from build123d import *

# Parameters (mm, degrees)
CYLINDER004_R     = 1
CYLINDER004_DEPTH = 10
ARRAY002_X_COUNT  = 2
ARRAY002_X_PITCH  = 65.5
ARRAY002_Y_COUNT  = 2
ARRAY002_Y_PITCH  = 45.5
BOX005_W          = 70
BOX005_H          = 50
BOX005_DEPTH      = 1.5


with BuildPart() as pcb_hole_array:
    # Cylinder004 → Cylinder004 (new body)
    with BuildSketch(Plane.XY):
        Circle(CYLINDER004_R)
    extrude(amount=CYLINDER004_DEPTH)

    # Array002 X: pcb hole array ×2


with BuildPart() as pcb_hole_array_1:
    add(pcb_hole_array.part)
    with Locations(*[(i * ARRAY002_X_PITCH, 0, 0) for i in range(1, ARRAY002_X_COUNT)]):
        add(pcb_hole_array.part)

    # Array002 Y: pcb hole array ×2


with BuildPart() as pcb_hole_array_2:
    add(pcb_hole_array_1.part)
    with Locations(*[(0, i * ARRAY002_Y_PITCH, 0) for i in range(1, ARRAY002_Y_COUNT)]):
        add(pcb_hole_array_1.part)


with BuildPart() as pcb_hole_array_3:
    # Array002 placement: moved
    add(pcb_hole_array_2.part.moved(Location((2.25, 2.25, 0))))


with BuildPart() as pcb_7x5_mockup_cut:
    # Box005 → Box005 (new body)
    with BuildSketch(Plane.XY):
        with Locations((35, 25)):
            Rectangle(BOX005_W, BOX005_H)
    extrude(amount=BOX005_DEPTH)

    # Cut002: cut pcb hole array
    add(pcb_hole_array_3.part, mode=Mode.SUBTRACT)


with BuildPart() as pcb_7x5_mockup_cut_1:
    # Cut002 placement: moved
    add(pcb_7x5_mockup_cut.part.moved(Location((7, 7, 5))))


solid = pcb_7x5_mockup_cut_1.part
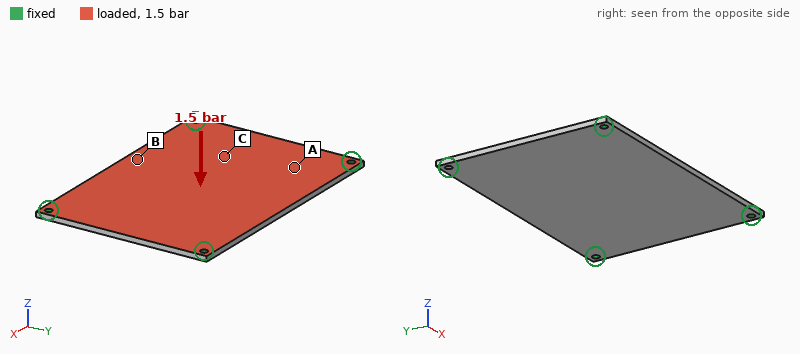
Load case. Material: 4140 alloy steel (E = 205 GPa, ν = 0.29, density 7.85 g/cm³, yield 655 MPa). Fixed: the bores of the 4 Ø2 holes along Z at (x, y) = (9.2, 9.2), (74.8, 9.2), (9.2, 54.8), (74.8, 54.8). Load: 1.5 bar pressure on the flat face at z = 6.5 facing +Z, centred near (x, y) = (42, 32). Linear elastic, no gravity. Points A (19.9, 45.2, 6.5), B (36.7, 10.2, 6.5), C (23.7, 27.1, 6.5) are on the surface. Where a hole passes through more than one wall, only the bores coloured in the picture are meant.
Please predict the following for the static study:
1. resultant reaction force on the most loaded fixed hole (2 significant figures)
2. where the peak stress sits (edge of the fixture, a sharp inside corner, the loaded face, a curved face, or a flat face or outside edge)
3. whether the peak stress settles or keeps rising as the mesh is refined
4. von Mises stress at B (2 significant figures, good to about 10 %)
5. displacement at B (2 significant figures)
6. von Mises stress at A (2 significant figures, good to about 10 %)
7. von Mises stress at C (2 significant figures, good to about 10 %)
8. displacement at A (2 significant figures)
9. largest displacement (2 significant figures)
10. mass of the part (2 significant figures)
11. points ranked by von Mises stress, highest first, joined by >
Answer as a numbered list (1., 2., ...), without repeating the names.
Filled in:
1. 130 N
2. edge of the fixture
3. keeps rising
4. 98 MPa
5. 0.20 mm
6. 32 MPa
7. 51 MPa
8. 0.10 mm
9. 0.24 mm
10. 41 g
11. B > C > A
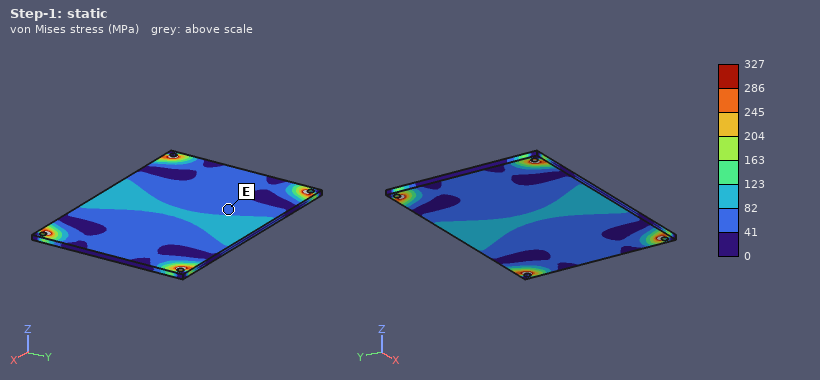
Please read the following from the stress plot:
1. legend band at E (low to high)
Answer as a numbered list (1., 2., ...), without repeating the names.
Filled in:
1. 41 to 82 MPa
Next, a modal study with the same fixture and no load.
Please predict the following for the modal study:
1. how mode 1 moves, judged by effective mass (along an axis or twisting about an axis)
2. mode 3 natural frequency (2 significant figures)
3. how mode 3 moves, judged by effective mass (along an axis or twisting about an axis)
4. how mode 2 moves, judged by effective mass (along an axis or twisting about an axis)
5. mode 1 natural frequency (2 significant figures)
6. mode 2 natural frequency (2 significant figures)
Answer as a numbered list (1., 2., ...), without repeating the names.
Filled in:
1. along Z
2. 3300 Hz
3. twisting about Y
4. twisting about X
5. 1400 Hz
6. 2400 Hz
